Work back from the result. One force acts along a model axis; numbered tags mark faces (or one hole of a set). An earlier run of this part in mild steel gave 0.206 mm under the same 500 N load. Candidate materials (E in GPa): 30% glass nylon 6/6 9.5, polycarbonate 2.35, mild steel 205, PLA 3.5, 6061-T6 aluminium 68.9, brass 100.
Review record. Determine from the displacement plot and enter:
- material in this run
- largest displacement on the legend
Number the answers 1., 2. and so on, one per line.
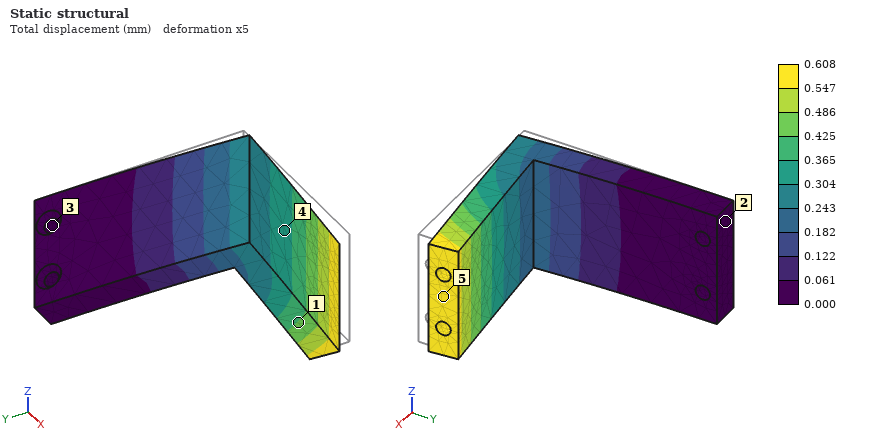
1. 6061-T6 aluminium
2. 0.608 mm
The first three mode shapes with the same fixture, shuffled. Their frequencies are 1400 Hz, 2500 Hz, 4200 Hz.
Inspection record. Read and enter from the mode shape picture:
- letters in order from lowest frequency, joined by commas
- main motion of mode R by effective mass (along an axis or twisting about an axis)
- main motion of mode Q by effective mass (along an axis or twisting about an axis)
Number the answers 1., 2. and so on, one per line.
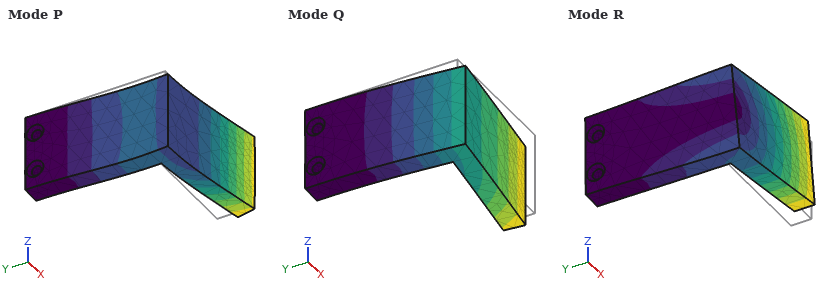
1. Q, R, P
2. along Z
3. along X
